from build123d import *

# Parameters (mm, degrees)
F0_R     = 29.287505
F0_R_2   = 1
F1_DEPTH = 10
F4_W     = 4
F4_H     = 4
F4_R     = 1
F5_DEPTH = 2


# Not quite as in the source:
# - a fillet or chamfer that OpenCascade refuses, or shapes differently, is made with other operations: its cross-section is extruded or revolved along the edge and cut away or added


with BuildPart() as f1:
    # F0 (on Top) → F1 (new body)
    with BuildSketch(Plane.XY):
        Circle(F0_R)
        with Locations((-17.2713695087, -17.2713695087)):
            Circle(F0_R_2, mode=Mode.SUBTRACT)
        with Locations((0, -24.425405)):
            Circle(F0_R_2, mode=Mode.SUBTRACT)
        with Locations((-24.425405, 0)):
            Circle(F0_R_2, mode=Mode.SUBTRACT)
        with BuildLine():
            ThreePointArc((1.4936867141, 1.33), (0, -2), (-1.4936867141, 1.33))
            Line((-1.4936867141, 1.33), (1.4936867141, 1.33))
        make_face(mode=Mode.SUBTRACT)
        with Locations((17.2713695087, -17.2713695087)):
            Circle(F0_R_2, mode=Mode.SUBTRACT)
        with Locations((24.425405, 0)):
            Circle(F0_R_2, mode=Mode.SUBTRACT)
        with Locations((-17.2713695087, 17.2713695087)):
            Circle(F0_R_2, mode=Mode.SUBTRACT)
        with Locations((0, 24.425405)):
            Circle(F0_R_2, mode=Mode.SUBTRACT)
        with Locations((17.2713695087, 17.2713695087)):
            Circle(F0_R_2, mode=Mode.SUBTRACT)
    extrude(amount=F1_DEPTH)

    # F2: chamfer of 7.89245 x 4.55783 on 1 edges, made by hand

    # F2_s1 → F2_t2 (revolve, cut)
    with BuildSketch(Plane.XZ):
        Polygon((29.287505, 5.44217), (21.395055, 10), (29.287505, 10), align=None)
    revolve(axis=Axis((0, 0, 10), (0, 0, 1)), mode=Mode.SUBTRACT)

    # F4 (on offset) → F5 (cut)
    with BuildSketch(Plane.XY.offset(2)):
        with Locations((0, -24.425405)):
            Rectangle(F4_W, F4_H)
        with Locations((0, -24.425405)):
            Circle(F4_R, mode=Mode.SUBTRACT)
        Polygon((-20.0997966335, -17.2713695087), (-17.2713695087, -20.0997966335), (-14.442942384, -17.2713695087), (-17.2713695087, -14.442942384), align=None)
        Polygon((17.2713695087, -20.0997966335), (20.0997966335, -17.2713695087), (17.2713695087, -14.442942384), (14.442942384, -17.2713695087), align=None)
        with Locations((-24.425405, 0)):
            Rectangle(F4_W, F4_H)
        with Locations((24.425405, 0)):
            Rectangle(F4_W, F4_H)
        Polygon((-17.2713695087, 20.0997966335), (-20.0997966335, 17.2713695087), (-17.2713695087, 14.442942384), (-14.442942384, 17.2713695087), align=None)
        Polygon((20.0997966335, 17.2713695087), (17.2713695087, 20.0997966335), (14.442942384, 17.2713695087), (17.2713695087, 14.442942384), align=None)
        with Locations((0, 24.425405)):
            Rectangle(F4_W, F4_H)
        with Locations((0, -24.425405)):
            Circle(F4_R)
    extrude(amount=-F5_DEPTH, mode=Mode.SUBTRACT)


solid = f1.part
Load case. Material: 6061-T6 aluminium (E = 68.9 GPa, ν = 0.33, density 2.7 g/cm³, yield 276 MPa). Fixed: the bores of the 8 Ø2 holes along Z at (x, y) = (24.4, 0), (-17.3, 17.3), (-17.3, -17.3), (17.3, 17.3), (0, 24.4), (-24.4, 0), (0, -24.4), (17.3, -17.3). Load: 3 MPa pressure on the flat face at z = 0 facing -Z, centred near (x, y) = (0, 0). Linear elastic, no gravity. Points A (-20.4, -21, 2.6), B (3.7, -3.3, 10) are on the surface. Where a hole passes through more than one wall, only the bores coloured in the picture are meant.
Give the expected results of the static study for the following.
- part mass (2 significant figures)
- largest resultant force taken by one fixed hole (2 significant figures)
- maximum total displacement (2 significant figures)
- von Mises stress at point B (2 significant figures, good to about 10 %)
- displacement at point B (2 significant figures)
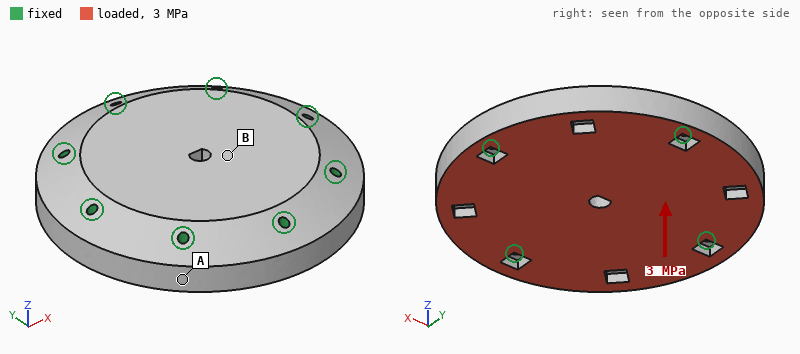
63 g
970 N
9.2 µm
14 MPa
8.3 µm
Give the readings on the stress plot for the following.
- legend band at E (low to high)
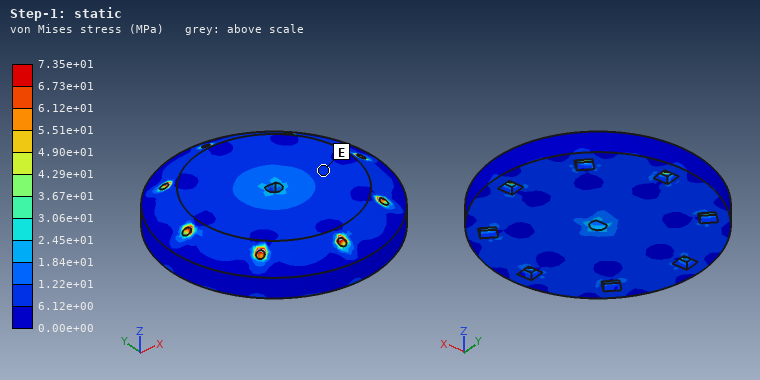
6.12e+00 to 1.22e+01 MPa
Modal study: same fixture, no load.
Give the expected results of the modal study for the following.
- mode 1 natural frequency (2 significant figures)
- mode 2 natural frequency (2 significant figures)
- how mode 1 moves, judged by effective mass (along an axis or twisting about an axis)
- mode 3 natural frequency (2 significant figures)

21 kHz
40 kHz
along Z
40 kHz
